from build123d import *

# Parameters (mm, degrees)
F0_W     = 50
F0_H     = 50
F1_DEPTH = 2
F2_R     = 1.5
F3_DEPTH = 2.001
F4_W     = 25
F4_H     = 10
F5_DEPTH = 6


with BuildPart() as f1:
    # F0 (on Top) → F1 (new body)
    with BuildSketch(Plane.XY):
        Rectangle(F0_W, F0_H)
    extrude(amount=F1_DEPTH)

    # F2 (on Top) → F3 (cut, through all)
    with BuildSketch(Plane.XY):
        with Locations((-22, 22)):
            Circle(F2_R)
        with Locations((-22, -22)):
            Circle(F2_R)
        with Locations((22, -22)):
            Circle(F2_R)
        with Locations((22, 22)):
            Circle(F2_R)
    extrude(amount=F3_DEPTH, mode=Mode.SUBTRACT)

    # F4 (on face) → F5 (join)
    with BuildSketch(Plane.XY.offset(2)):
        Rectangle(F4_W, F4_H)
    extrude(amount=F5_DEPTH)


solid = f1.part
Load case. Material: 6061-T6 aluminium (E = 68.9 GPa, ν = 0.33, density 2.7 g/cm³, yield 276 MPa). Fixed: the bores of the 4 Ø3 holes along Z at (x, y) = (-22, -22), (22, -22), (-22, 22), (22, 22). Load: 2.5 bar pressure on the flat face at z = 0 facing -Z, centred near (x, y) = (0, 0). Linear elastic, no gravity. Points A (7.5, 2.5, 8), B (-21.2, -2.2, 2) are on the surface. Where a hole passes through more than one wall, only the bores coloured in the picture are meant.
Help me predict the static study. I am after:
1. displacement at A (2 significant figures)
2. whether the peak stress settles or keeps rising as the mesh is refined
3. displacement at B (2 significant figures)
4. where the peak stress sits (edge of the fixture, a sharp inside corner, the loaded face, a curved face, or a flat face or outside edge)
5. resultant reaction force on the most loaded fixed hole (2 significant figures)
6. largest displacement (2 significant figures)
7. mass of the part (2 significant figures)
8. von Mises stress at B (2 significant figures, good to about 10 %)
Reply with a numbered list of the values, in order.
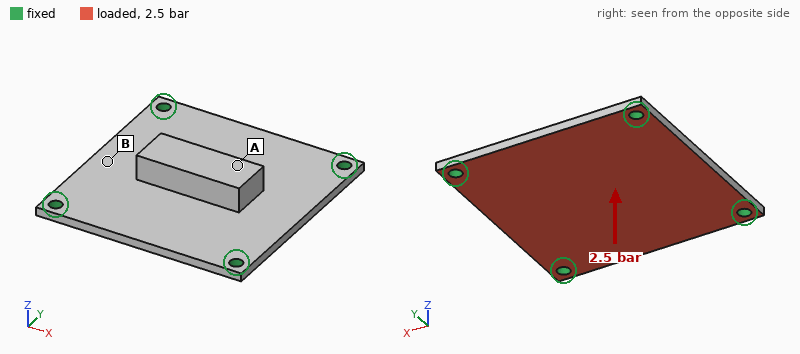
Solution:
1. 90 µm
2. keeps rising
3. 76 µm
4. edge of the fixture
5. 160 N
6. 91 µm
7. 17 g
8. 38 MPa
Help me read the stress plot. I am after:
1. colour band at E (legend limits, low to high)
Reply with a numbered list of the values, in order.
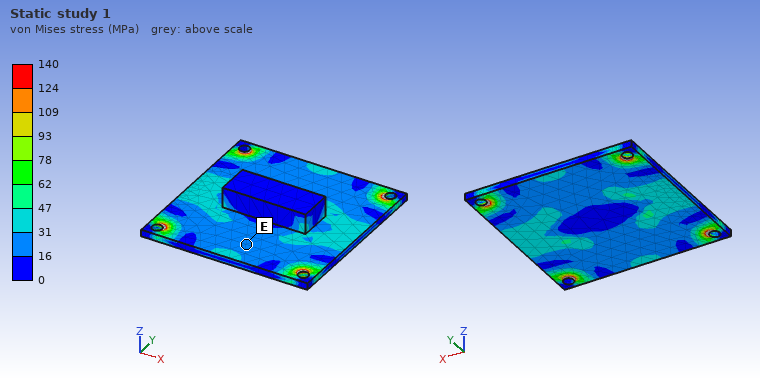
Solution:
1. 16 to 31 MPa
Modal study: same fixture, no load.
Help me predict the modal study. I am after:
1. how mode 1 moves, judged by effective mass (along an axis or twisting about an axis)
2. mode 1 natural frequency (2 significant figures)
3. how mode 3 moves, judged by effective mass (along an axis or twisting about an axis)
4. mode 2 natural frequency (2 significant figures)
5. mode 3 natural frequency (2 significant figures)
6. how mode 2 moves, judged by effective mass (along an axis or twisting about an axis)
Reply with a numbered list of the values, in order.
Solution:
1. along Z
2. 3200 Hz
3. twisting about X
4. 5600 Hz
5. 6100 Hz
6. twisting about Y
